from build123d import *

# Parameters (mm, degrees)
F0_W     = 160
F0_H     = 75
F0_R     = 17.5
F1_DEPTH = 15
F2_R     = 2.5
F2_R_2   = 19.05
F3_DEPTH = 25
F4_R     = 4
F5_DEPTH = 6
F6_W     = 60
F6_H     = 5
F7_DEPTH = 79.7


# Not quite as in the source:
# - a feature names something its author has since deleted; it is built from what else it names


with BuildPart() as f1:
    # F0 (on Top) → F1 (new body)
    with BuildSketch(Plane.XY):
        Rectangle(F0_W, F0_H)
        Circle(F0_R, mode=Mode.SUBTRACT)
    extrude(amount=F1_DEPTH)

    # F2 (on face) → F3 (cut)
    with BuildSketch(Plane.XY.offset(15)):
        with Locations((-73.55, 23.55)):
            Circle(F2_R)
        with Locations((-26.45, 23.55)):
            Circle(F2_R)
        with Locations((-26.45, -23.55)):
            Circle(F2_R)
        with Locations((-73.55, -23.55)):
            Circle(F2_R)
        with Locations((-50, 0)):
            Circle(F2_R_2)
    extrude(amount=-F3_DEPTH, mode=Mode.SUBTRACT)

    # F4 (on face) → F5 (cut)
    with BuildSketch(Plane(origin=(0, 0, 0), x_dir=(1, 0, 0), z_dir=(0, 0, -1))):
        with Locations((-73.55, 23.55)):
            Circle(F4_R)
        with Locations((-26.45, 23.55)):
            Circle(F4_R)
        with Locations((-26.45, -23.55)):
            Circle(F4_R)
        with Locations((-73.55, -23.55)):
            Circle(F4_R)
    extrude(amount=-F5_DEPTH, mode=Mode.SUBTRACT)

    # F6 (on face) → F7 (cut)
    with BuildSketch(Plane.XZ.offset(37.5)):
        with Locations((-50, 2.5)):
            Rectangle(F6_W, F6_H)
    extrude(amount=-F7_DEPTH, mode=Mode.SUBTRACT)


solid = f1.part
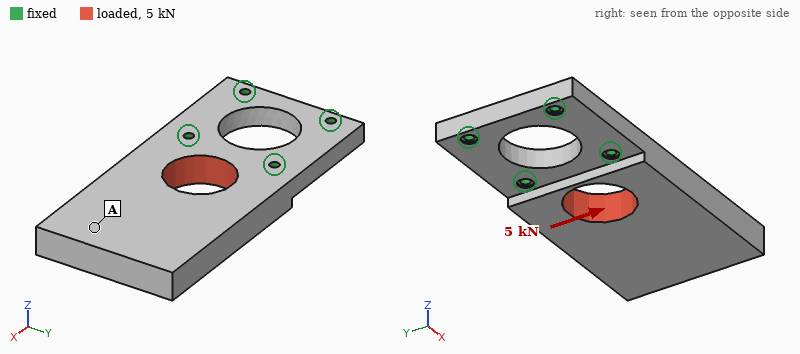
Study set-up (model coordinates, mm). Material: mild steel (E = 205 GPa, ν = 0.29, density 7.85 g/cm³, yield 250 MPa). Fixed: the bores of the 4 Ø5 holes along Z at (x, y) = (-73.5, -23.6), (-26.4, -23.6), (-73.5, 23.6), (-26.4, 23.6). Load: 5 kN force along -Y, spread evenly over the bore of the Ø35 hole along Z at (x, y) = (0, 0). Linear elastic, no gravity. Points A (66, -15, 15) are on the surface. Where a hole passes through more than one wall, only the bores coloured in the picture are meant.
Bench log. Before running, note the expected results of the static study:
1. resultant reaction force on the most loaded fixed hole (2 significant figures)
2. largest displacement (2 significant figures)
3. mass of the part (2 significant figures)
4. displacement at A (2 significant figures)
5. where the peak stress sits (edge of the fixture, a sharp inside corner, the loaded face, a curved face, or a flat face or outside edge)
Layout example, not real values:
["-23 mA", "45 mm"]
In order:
["3.2 kN", "13 µm", "1.0 kg", "12 µm", "edge of the fixture"]
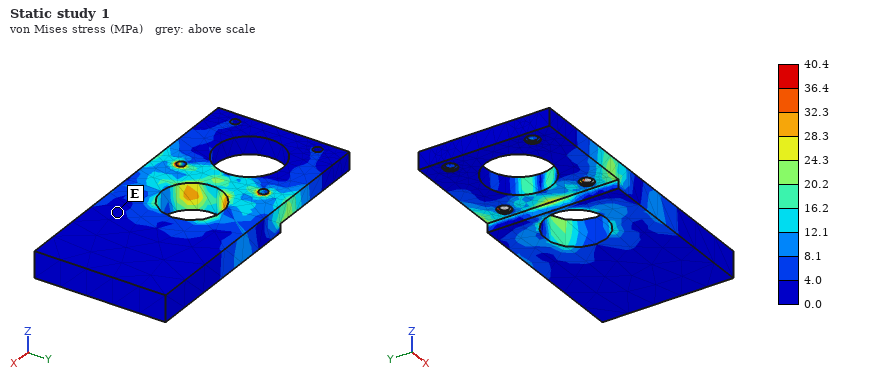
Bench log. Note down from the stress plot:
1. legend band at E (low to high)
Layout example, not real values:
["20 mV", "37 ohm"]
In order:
["0.0 to 4.0 MPa"]
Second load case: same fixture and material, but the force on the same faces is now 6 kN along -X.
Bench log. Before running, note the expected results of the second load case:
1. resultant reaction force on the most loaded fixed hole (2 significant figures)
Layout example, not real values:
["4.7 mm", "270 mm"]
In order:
["2.8 kN"]
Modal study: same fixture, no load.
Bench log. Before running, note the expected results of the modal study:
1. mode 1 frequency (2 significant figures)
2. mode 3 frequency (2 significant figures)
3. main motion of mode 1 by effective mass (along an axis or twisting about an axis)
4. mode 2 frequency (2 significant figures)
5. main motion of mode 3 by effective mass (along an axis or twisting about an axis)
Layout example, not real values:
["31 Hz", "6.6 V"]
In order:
["630 Hz", "2800 Hz", "along Z", "2400 Hz", "along Y"]
